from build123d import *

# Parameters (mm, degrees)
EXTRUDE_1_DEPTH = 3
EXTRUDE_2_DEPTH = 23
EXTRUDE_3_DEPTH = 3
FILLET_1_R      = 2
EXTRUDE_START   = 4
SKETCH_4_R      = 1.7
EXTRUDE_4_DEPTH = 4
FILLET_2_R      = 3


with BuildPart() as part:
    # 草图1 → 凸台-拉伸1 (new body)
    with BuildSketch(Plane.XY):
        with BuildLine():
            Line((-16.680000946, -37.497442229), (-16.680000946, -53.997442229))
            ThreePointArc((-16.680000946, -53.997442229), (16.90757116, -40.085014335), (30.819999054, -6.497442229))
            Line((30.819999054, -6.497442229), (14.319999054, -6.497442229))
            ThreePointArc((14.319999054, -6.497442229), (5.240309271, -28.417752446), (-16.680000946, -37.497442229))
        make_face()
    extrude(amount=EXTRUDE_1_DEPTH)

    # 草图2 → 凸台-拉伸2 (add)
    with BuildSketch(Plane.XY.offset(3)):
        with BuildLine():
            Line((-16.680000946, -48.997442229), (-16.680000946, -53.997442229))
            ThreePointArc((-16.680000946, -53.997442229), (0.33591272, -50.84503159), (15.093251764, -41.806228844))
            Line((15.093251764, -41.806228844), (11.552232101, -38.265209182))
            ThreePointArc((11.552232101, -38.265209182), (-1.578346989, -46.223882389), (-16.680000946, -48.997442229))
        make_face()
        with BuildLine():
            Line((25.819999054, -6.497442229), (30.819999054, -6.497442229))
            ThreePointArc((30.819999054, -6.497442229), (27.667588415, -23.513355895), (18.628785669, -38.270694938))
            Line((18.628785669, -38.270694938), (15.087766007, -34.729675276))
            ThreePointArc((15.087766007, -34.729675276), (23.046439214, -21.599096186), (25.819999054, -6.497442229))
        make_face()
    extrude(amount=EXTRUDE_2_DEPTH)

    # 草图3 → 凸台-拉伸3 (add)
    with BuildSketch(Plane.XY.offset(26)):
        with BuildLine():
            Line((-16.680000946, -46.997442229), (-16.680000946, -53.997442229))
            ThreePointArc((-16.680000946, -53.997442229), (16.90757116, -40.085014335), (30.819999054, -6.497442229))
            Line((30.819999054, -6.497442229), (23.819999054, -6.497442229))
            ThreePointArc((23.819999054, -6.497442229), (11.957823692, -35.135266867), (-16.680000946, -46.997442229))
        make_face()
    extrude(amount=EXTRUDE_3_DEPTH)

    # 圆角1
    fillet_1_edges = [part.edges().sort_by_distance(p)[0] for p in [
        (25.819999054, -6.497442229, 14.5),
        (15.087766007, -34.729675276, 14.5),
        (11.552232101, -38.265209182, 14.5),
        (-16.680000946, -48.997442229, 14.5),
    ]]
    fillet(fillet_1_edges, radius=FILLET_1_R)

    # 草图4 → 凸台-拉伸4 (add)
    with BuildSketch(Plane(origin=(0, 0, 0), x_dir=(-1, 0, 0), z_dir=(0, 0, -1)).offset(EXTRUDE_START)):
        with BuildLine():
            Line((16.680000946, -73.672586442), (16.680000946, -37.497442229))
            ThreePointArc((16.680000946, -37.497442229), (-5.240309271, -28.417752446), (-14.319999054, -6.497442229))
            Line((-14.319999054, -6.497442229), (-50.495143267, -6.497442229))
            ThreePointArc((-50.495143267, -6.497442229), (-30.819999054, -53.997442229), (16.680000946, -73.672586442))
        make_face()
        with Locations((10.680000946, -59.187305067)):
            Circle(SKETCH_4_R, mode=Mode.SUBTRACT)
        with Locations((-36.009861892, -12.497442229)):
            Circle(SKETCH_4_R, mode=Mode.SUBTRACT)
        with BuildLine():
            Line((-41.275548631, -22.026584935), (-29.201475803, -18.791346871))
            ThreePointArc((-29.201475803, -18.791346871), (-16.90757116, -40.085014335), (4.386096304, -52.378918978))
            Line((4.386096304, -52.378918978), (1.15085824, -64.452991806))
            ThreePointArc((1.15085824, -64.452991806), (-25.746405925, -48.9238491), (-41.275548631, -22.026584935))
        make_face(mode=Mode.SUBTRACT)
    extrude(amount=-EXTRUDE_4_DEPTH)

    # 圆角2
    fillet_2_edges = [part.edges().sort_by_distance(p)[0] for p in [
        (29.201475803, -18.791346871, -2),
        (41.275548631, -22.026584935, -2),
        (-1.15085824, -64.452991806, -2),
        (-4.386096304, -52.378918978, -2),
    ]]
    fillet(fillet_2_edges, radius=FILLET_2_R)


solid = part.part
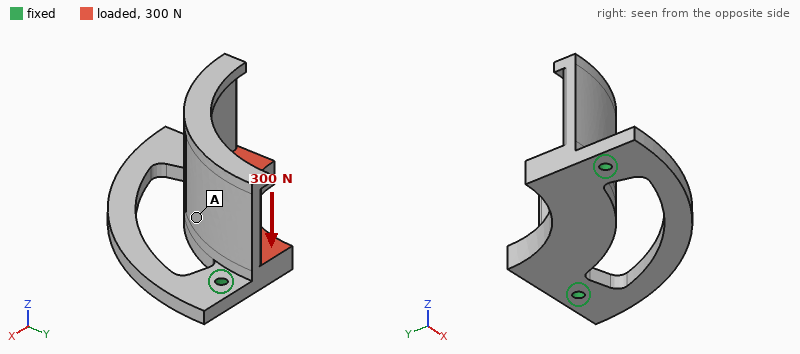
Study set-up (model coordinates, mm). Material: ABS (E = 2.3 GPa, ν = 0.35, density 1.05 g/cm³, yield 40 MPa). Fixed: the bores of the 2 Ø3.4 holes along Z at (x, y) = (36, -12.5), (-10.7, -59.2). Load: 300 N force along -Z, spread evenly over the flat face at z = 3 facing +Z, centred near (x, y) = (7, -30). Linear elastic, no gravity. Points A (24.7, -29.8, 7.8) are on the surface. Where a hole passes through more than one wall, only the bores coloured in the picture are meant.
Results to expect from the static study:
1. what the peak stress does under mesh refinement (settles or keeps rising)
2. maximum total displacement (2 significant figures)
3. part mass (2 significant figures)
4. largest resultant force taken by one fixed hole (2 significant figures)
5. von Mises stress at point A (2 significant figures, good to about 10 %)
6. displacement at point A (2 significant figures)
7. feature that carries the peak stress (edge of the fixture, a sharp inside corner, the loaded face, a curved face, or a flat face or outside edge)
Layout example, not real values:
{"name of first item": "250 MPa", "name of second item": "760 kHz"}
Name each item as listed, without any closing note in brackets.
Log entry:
{"what the peak stress does under mesh refinement": "keeps rising", "maximum total displacement": "0.73 mm", "part mass": "21 g", "largest resultant force taken by one fixed hole": "170 N", "von Mises stress at point A": "3.3 MPa", "displacement at point A": "0.23 mm", "feature that carries the peak stress": "edge of the fixture"}
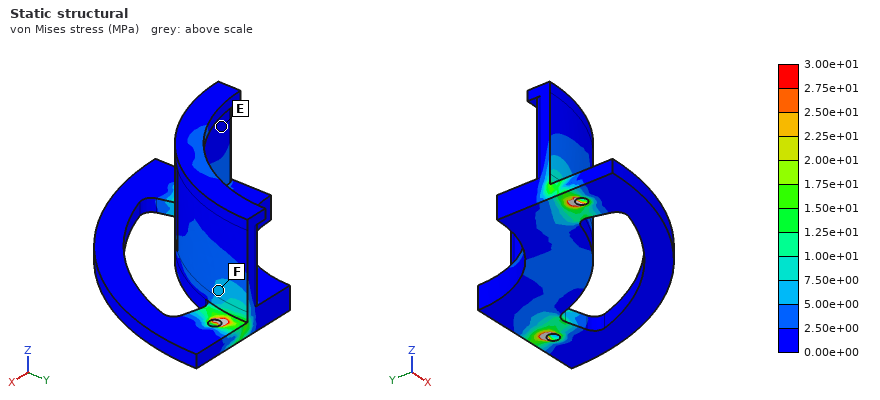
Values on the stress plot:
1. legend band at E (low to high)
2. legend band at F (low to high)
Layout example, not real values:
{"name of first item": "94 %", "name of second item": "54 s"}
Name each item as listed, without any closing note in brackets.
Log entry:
{"legend band at E": "0.00e+00 to 2.50e+00 MPa", "legend band at F": "5.00e+00 to 7.50e+00 MPa"}
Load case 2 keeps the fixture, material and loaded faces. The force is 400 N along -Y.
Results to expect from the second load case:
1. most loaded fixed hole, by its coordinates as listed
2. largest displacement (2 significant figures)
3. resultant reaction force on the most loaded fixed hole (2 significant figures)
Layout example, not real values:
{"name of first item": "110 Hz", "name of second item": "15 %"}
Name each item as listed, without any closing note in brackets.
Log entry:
{"most loaded fixed hole, by its coordinates as listed": "(-10.7, -59.2)", "largest displacement": "0.83 mm", "resultant reaction force on the most loaded fixed hole": "260 N"}
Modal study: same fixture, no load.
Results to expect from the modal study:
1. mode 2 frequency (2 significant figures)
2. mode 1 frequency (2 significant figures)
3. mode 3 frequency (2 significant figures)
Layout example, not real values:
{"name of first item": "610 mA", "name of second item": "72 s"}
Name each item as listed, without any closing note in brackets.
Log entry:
{"mode 2 frequency": "820 Hz", "mode 1 frequency": "560 Hz", "mode 3 frequency": "1400 Hz"}
